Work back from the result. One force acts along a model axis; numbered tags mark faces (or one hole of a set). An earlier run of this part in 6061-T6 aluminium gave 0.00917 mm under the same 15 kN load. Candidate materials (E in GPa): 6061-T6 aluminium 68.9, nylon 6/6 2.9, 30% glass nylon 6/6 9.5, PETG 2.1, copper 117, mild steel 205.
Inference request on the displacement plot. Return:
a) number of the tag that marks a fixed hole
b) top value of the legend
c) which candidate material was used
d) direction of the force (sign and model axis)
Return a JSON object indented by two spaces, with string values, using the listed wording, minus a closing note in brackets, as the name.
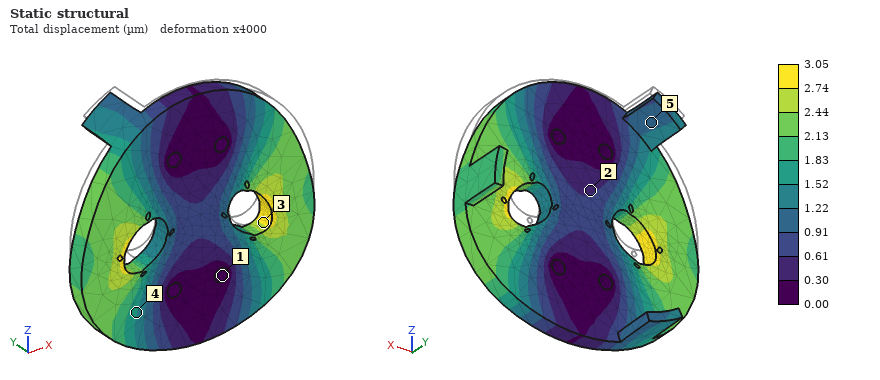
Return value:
{
  "number of the tag that marks a fixed hole": "1",
  "top value of the legend": "3.05 µm",
  "which candidate material was used": "mild steel",
  "direction of the force": "-Z"
}
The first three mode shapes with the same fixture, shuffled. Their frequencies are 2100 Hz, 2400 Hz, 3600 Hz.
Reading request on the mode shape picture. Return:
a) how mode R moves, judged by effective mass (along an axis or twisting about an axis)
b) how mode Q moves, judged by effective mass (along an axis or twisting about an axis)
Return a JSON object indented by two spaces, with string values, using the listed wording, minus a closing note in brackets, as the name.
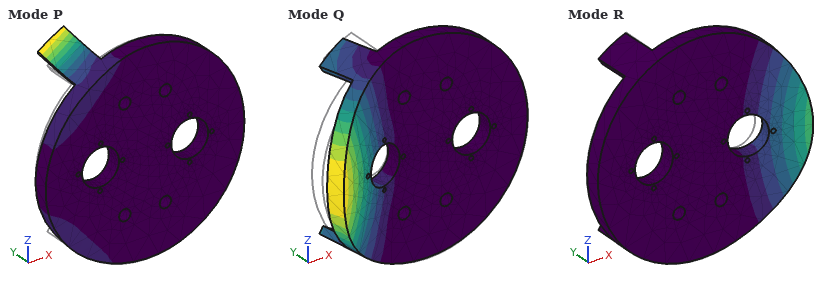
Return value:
{
  "how mode R moves, judged by effective mass": "along Y",
  "how mode Q moves, judged by effective mass": "along Y"
}
